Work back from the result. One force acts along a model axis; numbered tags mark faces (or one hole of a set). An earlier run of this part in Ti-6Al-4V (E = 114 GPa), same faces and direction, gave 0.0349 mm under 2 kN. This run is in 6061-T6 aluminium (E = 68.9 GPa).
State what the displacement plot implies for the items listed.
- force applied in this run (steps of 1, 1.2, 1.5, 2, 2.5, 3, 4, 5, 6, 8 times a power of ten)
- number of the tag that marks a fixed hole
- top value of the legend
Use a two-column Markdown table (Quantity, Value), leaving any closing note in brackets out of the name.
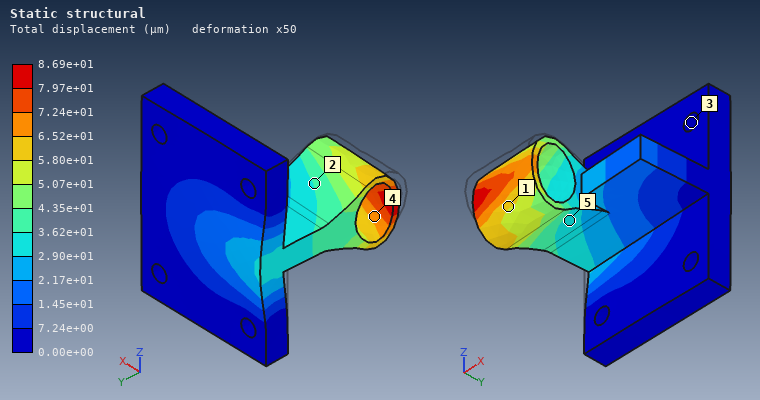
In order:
| Quantity | Value |
|---|---|
| force applied in this run | 3 kN |
| number of the tag that marks a fixed hole | 3 |
| top value of the legend | 8.69e+01 µm |
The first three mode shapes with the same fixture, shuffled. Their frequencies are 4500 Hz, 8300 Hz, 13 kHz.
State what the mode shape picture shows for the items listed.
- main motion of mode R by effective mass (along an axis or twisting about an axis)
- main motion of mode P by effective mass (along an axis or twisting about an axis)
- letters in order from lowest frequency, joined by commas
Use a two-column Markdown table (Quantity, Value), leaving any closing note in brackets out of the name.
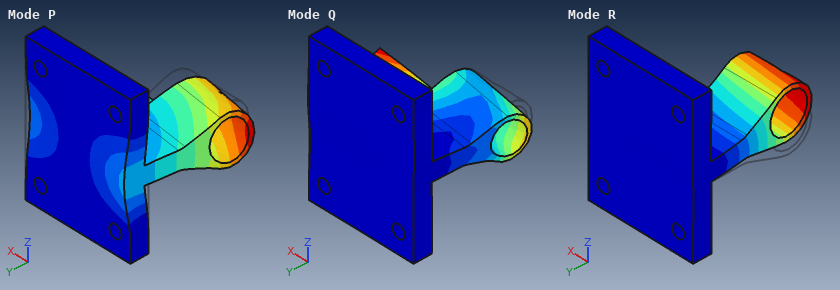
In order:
| Quantity | Value |
|---|---|
| main motion of mode R by effective mass | along Z |
| main motion of mode P by effective mass | along X |
| letters in order from lowest frequency, joined by commas | R, P, Q |
